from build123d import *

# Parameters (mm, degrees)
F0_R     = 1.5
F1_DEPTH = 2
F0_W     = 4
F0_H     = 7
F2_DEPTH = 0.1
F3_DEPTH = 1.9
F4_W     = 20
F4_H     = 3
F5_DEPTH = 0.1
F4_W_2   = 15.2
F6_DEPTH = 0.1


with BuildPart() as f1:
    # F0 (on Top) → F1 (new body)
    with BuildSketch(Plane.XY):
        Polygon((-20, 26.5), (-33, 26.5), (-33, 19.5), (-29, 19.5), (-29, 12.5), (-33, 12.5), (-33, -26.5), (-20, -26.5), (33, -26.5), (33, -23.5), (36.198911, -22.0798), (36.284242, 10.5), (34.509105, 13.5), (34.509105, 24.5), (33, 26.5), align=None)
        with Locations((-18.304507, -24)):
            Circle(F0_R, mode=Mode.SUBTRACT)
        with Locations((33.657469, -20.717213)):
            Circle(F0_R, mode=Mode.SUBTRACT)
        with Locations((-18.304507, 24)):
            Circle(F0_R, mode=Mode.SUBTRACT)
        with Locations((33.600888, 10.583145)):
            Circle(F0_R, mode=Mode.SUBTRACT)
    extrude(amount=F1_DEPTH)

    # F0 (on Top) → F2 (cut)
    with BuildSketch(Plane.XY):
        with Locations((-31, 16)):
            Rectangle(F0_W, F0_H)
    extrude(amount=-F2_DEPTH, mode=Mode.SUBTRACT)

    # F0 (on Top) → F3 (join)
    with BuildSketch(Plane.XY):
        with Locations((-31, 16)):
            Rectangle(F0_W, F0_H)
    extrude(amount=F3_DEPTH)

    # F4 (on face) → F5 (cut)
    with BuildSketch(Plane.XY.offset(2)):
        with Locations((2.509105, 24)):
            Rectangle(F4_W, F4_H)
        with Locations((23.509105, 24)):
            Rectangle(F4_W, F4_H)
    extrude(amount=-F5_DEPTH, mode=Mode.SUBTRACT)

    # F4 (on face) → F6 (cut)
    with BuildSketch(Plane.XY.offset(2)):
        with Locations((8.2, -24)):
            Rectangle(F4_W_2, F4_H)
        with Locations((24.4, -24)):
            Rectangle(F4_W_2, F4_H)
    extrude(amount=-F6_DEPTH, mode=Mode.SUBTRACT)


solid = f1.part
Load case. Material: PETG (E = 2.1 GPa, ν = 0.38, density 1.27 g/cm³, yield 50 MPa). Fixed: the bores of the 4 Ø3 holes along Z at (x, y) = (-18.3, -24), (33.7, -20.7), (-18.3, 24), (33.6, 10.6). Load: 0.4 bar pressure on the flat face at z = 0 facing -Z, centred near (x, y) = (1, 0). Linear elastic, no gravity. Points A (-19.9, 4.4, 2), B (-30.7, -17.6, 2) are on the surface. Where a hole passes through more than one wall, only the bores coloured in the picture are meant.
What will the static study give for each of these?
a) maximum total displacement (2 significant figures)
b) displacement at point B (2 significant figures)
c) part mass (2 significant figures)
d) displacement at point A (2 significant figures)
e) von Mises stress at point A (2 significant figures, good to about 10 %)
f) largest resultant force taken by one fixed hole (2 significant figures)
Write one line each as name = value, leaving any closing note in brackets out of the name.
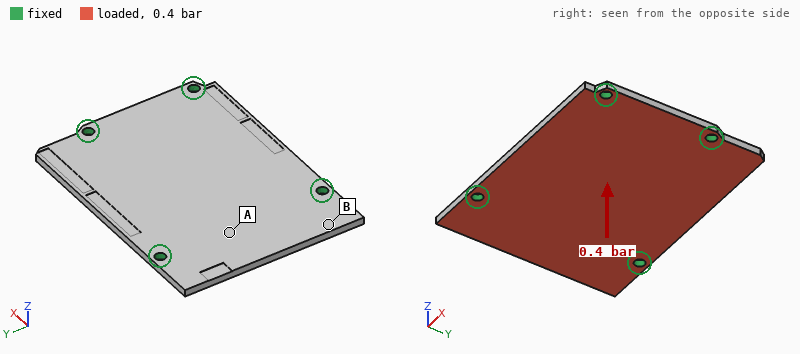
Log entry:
maximum total displacement = 0.89 mm
displacement at point B = 0.22 mm
part mass = 9.1 g
displacement at point A = 0.54 mm
von Mises stress at point A = 6.8 MPa
largest resultant force taken by one fixed hole = 43 N
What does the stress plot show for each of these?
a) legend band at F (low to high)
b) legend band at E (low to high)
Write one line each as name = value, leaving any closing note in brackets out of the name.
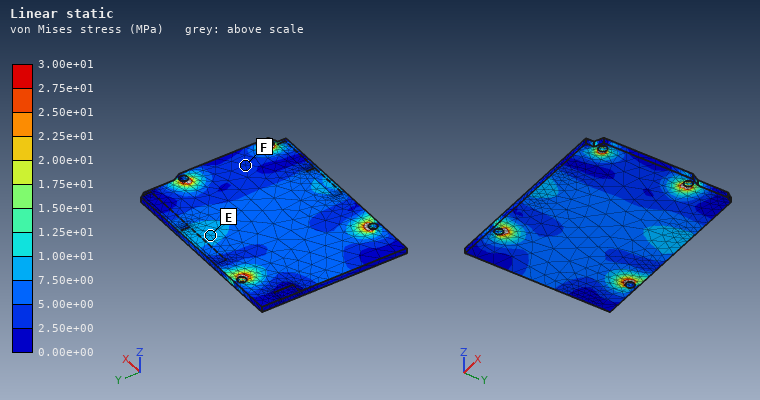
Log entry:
legend band at F = 2.50e+00 to 5.00e+00 MPa
legend band at E = 7.50e+00 to 1.00e+01 MPa
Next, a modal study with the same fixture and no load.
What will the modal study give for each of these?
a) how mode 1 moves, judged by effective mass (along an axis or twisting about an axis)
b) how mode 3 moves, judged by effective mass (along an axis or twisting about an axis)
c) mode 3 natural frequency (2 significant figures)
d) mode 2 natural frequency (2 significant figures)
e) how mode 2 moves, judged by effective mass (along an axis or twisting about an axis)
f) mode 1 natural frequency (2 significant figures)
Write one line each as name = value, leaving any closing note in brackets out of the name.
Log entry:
how mode 1 moves, judged by effective mass = along Z
how mode 3 moves, judged by effective mass = twisting about X
mode 3 natural frequency = 1000 Hz
mode 2 natural frequency = 950 Hz
how mode 2 moves, judged by effective mass = along Z
mode 1 natural frequency = 770 Hz
